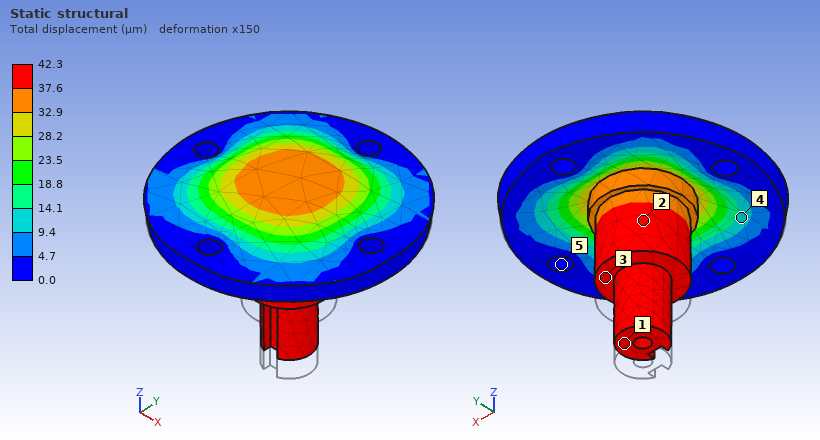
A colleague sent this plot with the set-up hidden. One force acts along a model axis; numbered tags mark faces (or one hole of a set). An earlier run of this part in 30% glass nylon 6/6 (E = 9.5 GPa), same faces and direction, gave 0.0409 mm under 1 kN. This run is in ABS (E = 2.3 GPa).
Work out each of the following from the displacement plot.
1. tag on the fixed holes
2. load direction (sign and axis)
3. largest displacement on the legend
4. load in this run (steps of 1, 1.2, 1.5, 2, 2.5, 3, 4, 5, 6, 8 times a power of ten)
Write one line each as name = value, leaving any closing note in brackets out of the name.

tag on the fixed holes = 5
load direction = +Z
largest displacement on the legend = 42.3 µm
load in this run = 250 N
